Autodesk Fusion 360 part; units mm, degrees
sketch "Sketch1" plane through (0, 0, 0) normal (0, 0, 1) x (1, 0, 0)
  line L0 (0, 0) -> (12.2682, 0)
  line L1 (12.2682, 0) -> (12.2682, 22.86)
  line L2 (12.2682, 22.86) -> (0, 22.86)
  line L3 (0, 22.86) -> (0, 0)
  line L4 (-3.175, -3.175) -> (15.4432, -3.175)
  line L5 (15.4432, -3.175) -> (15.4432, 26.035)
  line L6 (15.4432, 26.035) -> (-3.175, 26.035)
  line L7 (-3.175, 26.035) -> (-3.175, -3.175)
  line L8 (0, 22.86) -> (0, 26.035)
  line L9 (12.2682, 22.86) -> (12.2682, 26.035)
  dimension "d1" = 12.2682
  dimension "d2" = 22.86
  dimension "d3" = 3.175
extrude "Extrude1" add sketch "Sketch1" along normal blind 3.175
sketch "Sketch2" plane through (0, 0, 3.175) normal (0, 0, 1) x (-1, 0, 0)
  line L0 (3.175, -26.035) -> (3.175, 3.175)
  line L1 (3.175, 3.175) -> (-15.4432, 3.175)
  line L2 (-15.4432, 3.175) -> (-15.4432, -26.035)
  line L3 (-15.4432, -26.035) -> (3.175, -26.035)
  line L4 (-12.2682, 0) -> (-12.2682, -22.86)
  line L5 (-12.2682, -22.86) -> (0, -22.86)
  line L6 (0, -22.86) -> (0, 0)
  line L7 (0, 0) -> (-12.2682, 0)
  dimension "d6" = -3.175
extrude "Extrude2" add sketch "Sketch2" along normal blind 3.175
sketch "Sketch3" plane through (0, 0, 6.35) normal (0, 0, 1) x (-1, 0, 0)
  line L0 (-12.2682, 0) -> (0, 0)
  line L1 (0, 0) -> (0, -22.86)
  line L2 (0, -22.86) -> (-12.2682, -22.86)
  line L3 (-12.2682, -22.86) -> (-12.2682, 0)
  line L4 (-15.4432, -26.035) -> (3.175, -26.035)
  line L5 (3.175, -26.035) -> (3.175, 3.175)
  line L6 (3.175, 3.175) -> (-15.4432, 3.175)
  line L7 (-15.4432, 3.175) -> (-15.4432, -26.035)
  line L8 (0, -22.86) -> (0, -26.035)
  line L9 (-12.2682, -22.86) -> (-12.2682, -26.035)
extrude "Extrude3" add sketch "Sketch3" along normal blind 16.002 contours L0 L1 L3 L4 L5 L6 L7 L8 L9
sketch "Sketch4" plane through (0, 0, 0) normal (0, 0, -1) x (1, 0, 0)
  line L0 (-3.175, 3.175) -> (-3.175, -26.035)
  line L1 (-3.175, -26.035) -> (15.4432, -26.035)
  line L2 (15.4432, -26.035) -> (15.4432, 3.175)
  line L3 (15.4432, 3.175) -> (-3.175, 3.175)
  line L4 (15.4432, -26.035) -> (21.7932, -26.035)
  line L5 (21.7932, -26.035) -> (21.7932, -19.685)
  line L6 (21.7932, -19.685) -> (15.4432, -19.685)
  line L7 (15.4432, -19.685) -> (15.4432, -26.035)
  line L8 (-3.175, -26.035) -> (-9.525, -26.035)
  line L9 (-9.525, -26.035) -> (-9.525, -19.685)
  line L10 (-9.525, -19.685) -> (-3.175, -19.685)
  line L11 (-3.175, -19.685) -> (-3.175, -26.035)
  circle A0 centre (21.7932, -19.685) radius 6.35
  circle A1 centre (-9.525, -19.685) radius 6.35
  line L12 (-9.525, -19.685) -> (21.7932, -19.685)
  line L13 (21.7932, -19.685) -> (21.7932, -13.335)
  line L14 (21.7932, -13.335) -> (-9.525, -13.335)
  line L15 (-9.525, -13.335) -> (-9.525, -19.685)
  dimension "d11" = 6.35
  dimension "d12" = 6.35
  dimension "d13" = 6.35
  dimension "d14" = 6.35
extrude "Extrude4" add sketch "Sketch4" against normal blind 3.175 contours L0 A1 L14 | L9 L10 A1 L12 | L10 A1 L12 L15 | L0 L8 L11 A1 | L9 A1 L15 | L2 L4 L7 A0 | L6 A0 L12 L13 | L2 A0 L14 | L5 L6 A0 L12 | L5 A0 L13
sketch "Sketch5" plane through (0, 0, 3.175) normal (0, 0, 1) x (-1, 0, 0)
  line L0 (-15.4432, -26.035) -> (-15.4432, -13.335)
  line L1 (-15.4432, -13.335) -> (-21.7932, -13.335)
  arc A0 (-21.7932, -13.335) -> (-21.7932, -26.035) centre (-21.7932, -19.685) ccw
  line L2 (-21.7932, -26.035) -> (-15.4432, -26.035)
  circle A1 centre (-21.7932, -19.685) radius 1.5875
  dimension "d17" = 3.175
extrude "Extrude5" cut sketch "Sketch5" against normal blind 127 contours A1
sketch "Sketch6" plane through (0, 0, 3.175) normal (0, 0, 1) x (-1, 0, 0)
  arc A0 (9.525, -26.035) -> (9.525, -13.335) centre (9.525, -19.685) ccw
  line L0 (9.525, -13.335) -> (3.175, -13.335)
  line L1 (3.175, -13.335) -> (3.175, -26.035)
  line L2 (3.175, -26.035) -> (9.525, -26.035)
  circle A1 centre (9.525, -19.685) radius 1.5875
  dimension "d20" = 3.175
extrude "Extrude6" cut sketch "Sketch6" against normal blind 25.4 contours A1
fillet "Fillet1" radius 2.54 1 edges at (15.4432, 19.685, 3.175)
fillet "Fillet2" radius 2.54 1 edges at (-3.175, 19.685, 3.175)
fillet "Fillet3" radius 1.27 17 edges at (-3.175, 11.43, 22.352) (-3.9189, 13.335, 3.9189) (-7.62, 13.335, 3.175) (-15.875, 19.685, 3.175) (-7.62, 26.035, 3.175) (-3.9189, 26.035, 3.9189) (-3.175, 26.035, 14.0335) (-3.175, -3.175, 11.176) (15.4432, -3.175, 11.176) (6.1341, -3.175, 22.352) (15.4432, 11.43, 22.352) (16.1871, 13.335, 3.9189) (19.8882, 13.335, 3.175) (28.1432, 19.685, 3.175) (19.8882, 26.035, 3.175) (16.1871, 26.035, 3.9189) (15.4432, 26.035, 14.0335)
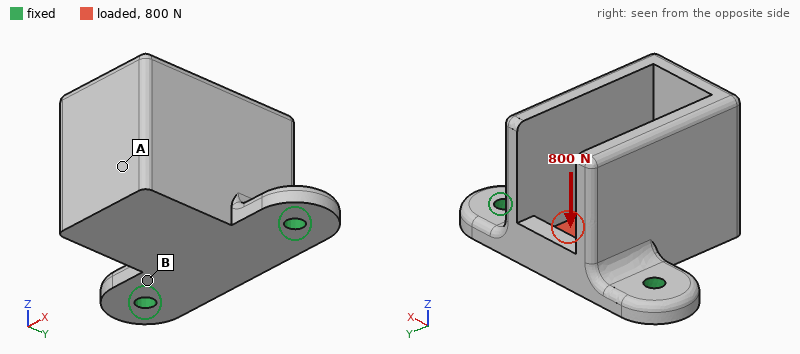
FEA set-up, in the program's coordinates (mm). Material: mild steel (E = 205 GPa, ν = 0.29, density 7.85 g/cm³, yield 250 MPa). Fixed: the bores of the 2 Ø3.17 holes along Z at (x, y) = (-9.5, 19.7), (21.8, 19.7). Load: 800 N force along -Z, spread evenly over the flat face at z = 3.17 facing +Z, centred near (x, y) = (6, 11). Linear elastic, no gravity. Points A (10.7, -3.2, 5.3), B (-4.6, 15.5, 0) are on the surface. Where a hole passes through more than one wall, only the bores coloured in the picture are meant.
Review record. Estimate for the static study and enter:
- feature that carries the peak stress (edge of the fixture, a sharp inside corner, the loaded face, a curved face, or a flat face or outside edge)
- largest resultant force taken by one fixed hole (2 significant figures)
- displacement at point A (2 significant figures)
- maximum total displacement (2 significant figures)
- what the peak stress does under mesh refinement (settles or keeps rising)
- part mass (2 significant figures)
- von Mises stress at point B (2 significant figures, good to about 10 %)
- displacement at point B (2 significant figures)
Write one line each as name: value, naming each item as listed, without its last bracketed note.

feature that carries the peak stress: edge of the fixture
largest resultant force taken by one fixed hole: 430 N
displacement at point A: 46 µm
maximum total displacement: 58 µm
what the peak stress does under mesh refinement: keeps rising
part mass: 55 g
von Mises stress at point B: 73 MPa
displacement at point B: 8.7 µm
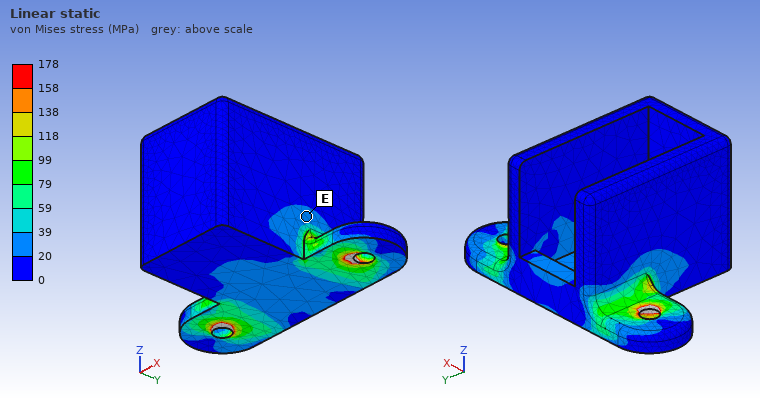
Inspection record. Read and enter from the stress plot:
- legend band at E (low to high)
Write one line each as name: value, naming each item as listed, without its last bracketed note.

legend band at E: 20 to 39 MPa
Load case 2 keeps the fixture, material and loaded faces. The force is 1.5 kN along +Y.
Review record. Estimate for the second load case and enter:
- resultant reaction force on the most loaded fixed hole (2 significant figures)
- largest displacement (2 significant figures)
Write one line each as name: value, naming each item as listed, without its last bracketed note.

resultant reaction force on the most loaded fixed hole: 760 N
largest displacement: 21 µm
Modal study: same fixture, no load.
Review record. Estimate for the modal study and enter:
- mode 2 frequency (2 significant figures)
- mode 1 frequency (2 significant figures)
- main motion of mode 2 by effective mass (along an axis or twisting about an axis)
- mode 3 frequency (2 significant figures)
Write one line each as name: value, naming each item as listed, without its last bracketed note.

mode 2 frequency: 5500 Hz
mode 1 frequency: 2600 Hz
main motion of mode 2 by effective mass: along X
mode 3 frequency: 8600 Hz
